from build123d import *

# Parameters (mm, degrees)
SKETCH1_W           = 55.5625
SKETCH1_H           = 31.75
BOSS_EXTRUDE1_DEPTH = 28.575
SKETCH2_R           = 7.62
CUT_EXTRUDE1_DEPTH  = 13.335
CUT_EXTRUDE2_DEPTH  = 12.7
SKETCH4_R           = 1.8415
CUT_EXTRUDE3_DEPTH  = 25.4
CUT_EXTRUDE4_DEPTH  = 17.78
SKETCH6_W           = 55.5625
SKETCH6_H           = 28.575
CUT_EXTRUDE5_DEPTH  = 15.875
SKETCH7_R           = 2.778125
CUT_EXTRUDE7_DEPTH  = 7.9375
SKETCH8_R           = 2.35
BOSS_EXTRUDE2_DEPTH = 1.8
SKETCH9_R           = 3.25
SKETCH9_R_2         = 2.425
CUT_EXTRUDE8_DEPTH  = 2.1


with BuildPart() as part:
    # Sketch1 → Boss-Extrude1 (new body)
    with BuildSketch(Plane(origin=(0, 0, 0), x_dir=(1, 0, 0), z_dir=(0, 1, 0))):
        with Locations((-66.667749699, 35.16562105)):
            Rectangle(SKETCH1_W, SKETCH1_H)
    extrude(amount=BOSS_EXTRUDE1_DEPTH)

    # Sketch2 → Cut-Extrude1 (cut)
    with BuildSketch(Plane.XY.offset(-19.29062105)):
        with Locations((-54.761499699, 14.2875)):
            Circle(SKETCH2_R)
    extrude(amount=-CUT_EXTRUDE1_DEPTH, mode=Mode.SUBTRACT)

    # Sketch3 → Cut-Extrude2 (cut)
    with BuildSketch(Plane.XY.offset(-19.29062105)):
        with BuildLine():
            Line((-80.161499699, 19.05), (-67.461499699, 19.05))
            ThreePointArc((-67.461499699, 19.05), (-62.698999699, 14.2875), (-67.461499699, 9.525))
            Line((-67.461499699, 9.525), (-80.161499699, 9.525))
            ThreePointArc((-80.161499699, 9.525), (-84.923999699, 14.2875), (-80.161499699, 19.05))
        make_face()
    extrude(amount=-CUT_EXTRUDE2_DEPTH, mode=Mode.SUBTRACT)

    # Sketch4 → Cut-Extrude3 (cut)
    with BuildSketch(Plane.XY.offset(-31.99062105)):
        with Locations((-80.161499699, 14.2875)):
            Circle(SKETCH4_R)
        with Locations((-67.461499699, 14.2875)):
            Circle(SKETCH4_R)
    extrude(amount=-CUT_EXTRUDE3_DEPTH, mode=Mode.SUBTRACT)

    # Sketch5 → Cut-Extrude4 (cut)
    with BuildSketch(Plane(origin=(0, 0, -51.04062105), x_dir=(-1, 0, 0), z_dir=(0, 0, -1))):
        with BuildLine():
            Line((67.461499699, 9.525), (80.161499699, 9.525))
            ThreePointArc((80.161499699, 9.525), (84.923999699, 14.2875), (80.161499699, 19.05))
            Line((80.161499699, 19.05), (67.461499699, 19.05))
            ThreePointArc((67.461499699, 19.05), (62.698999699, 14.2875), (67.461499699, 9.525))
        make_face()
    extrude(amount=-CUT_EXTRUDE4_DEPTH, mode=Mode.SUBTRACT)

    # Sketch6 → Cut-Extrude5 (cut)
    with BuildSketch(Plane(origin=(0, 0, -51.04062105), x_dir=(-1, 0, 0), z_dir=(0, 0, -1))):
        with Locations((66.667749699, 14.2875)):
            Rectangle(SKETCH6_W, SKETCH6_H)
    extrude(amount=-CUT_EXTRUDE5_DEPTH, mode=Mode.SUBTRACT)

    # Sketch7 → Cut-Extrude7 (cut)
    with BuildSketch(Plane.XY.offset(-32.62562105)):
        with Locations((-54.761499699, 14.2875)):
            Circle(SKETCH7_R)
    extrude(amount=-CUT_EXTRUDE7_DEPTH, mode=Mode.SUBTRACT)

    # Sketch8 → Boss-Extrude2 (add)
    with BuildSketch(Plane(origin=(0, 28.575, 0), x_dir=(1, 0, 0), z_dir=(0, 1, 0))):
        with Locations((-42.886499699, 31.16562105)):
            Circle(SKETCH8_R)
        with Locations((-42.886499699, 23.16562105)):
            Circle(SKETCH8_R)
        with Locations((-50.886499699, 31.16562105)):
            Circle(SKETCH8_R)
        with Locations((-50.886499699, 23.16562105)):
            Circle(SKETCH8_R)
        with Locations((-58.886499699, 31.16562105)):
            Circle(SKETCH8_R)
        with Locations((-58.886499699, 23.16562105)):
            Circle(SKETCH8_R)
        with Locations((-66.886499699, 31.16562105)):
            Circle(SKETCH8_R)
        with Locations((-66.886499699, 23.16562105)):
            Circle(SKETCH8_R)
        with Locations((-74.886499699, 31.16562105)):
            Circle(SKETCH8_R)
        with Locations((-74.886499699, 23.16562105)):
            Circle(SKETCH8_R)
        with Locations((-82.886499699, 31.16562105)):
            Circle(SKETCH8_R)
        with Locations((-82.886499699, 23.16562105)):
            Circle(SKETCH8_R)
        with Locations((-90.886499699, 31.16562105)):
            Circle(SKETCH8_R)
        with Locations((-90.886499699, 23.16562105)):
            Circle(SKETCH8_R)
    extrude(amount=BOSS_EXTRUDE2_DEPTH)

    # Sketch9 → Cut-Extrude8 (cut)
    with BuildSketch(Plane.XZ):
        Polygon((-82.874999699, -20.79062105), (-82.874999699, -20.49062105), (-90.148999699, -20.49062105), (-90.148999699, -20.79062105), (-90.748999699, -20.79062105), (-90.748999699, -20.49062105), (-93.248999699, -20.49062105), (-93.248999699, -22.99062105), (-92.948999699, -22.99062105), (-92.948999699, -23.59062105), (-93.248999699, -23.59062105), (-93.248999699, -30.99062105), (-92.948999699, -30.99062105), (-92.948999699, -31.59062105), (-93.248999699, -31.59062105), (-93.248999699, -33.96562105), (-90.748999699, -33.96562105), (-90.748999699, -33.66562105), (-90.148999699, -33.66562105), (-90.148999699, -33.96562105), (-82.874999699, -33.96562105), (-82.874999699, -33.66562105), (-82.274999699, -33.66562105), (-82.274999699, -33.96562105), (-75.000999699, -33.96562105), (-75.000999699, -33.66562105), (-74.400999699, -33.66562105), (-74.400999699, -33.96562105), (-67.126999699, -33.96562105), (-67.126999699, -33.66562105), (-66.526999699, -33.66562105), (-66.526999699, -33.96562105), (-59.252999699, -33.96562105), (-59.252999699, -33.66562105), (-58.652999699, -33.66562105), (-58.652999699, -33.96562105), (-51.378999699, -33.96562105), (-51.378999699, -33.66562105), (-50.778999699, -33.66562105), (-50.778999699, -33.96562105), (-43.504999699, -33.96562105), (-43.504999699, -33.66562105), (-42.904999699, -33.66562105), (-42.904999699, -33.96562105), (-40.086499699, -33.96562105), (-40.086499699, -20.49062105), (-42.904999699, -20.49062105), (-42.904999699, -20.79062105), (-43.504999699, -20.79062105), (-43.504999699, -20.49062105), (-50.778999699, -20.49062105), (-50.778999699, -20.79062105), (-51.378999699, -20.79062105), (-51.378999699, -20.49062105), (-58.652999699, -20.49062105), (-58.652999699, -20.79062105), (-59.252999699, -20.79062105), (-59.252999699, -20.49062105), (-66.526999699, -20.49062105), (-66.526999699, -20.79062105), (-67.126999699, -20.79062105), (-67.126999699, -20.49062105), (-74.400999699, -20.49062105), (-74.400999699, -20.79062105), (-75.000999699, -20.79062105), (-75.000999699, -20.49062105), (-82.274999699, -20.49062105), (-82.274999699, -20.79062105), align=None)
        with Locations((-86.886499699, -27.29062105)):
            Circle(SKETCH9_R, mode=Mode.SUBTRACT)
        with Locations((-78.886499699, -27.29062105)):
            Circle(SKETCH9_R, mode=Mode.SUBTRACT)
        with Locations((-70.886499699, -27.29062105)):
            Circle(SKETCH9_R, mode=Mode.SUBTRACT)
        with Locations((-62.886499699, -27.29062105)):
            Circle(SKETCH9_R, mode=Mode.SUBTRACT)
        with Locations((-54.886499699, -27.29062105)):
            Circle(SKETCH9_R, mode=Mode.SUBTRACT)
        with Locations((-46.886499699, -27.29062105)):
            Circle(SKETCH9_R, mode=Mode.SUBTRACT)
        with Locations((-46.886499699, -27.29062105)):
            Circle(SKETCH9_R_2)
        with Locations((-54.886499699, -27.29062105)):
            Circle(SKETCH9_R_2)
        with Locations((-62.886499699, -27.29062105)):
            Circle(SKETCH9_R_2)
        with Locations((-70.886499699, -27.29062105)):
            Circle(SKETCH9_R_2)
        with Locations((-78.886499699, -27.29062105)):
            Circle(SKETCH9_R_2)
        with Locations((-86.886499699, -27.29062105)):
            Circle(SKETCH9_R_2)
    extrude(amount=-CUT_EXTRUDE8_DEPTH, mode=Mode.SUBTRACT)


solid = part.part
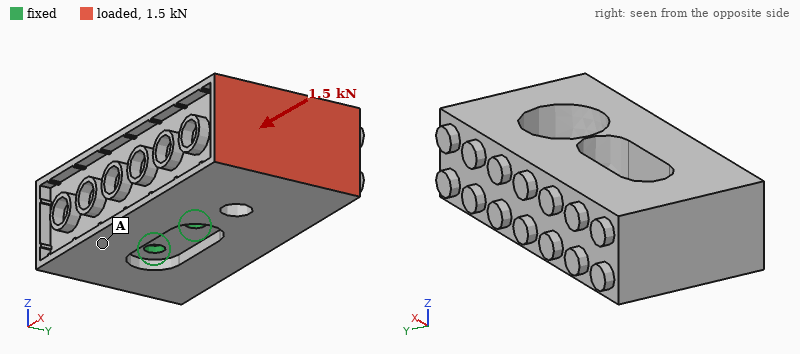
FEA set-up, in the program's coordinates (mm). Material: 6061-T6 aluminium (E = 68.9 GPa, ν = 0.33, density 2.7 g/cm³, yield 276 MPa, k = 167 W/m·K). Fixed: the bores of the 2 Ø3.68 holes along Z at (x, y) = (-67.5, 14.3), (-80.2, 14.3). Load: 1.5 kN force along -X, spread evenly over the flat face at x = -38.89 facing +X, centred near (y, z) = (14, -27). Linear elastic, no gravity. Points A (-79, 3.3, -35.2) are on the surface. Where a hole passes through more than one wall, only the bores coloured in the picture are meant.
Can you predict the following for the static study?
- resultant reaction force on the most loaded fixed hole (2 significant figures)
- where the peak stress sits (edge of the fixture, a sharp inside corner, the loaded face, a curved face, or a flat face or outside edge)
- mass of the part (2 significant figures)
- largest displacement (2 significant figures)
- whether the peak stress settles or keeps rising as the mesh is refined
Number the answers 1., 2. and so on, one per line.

1. 930 N
2. edge of the fixture
3. 51 g
4. 61 µm
5. keeps rising
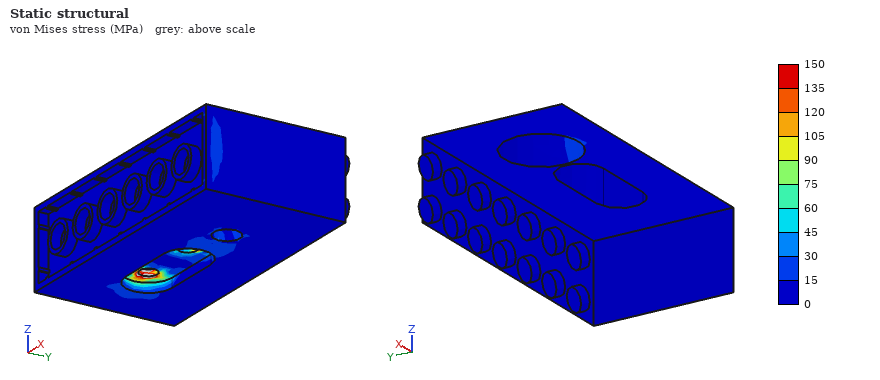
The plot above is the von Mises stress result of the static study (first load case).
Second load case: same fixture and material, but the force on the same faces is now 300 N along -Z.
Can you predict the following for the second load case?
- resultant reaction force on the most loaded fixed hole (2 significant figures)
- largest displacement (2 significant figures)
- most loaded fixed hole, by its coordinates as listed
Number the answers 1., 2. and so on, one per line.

1. 810 N
2. 85 µm
3. (-67.5, 14.3)
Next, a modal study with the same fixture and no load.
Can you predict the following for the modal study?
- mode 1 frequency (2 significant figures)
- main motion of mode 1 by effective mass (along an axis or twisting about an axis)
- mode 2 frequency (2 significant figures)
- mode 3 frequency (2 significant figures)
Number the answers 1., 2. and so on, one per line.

1. 1700 Hz
2. along Y
3. 2500 Hz
4. 4800 Hz
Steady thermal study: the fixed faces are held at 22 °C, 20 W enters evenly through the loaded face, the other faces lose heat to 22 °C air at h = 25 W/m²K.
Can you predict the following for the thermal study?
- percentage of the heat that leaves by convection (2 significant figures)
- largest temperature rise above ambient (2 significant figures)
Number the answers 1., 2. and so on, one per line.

1. 11 %
2. 22 K
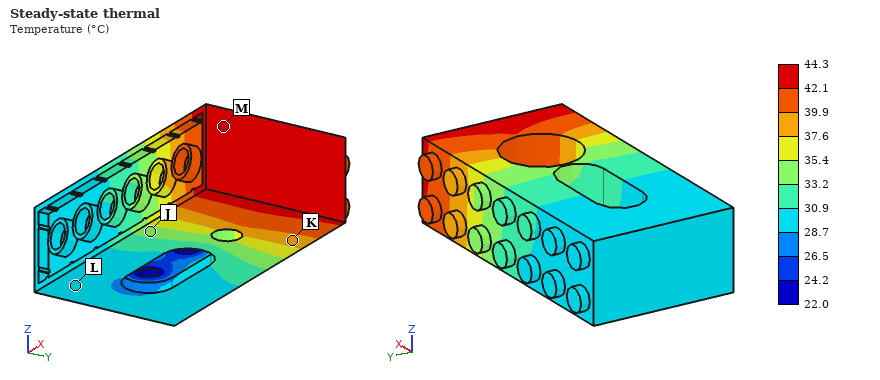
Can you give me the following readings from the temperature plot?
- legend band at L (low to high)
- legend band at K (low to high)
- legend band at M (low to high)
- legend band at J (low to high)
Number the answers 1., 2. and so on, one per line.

1. 28.7 to 30.9 °C
2. 37.6 to 39.9 °C
3. 42.1 to 44.3 °C
4. 33.2 to 35.4 °C
